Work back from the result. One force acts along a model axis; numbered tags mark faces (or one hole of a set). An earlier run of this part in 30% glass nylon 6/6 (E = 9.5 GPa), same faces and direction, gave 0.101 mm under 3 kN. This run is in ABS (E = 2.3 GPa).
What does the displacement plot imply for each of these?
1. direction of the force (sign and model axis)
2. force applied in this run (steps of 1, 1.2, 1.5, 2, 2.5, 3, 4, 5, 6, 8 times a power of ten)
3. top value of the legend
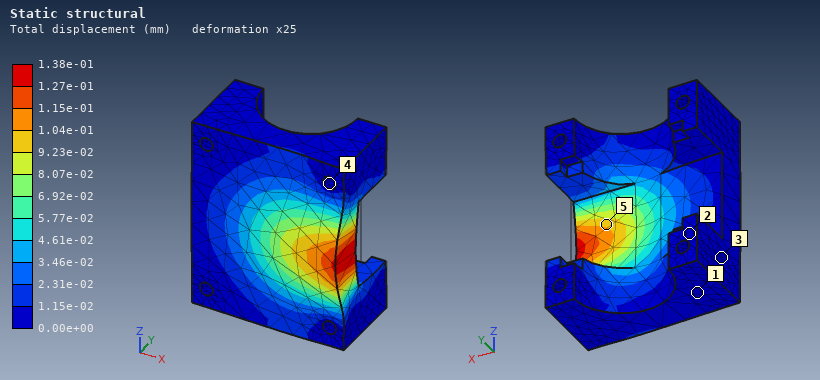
-Y
1 kN
1.38e-01 mm
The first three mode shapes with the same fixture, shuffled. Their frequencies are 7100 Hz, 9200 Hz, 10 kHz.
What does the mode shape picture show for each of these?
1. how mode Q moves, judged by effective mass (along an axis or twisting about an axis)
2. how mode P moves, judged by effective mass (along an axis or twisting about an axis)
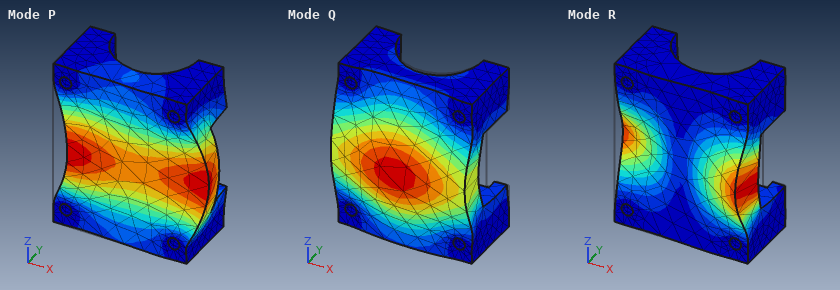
along Y
along X
